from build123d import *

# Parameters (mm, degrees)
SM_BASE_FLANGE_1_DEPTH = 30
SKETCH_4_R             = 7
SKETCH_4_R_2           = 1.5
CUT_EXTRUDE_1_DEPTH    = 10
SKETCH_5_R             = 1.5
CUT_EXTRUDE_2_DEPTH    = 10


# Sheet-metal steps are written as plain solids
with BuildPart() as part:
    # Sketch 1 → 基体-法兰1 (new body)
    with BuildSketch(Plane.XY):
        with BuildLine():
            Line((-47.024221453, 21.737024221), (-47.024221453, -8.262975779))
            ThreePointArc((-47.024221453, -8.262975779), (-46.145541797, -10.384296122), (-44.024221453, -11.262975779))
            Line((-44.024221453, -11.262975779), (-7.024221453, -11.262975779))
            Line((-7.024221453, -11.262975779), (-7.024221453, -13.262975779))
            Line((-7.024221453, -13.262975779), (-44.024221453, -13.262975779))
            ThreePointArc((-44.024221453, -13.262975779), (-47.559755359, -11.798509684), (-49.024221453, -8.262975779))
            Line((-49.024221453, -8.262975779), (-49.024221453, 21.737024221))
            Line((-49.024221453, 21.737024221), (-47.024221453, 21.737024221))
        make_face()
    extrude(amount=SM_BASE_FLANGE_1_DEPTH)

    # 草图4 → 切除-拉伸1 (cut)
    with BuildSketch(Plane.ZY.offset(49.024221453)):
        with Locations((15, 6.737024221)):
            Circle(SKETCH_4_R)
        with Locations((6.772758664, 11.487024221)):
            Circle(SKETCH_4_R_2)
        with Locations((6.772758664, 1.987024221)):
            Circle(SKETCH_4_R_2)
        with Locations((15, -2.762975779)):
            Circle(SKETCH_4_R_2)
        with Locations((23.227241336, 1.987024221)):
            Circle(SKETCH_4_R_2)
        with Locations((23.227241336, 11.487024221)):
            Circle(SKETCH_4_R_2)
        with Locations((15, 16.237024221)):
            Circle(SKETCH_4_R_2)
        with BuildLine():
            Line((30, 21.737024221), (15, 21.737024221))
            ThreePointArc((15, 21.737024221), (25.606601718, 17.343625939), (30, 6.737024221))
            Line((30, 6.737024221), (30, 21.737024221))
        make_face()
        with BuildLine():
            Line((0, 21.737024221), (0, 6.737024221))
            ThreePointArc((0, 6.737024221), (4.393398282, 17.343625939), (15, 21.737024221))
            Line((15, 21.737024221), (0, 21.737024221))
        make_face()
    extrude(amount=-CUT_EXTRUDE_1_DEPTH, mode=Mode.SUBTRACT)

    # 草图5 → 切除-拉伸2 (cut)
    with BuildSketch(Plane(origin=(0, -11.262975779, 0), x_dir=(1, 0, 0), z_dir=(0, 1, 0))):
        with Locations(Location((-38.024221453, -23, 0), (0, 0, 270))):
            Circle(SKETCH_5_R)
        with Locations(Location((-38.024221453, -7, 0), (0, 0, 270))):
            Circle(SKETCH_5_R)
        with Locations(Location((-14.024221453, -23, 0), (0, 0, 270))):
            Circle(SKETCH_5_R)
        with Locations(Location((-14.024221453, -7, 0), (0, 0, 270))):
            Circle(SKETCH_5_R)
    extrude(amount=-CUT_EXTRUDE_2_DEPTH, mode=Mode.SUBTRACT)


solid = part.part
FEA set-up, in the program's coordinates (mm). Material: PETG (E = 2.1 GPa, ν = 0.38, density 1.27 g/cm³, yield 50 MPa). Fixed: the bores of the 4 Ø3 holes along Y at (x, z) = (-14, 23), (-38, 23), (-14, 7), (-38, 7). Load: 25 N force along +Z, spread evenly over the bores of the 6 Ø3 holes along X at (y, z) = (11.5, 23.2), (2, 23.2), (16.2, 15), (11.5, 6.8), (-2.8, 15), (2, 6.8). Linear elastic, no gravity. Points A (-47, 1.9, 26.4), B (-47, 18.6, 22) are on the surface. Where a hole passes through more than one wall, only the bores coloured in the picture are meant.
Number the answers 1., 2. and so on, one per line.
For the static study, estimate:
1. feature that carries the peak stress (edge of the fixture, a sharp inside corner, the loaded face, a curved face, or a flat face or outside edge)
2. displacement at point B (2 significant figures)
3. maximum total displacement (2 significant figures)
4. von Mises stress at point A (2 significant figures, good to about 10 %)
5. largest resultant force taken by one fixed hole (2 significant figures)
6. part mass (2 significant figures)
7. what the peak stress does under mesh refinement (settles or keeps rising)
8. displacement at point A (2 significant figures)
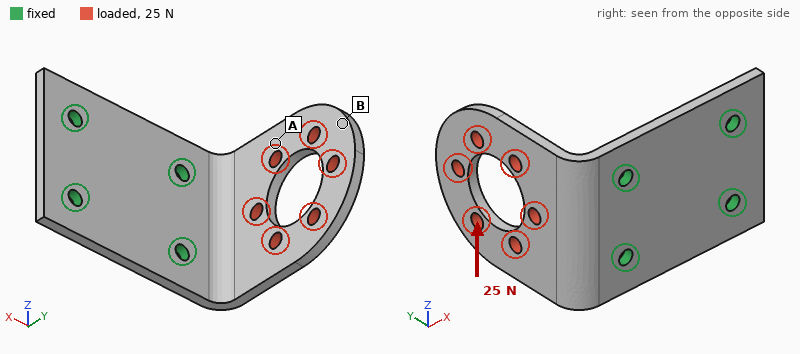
1. edge of the fixture
2. 0.71 mm
3. 0.74 mm
4. 3.2 MPa
5. 31 N
6. 4.8 g
7. keeps rising
8. 0.43 mm
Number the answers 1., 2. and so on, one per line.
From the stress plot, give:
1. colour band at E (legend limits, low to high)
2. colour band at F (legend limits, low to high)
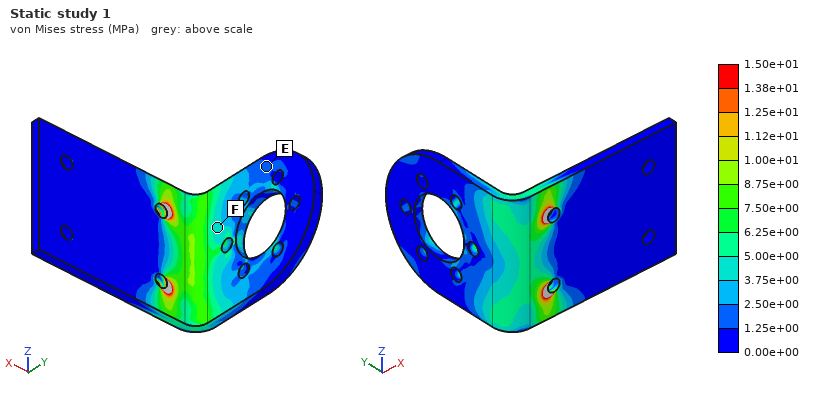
1. 1.25e+00 to 2.50e+00 MPa
2. 3.75e+00 to 5.00e+00 MPa
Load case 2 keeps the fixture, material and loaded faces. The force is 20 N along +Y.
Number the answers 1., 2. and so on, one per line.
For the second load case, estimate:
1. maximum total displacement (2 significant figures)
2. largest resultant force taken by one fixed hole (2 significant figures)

1. 0.75 mm
2. 11 N
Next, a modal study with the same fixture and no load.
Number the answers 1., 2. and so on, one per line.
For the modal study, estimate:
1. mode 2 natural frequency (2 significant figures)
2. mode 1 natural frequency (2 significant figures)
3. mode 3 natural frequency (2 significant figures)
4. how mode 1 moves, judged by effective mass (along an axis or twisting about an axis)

1. 780 Hz
2. 330 Hz
3. 1200 Hz
4. along X
